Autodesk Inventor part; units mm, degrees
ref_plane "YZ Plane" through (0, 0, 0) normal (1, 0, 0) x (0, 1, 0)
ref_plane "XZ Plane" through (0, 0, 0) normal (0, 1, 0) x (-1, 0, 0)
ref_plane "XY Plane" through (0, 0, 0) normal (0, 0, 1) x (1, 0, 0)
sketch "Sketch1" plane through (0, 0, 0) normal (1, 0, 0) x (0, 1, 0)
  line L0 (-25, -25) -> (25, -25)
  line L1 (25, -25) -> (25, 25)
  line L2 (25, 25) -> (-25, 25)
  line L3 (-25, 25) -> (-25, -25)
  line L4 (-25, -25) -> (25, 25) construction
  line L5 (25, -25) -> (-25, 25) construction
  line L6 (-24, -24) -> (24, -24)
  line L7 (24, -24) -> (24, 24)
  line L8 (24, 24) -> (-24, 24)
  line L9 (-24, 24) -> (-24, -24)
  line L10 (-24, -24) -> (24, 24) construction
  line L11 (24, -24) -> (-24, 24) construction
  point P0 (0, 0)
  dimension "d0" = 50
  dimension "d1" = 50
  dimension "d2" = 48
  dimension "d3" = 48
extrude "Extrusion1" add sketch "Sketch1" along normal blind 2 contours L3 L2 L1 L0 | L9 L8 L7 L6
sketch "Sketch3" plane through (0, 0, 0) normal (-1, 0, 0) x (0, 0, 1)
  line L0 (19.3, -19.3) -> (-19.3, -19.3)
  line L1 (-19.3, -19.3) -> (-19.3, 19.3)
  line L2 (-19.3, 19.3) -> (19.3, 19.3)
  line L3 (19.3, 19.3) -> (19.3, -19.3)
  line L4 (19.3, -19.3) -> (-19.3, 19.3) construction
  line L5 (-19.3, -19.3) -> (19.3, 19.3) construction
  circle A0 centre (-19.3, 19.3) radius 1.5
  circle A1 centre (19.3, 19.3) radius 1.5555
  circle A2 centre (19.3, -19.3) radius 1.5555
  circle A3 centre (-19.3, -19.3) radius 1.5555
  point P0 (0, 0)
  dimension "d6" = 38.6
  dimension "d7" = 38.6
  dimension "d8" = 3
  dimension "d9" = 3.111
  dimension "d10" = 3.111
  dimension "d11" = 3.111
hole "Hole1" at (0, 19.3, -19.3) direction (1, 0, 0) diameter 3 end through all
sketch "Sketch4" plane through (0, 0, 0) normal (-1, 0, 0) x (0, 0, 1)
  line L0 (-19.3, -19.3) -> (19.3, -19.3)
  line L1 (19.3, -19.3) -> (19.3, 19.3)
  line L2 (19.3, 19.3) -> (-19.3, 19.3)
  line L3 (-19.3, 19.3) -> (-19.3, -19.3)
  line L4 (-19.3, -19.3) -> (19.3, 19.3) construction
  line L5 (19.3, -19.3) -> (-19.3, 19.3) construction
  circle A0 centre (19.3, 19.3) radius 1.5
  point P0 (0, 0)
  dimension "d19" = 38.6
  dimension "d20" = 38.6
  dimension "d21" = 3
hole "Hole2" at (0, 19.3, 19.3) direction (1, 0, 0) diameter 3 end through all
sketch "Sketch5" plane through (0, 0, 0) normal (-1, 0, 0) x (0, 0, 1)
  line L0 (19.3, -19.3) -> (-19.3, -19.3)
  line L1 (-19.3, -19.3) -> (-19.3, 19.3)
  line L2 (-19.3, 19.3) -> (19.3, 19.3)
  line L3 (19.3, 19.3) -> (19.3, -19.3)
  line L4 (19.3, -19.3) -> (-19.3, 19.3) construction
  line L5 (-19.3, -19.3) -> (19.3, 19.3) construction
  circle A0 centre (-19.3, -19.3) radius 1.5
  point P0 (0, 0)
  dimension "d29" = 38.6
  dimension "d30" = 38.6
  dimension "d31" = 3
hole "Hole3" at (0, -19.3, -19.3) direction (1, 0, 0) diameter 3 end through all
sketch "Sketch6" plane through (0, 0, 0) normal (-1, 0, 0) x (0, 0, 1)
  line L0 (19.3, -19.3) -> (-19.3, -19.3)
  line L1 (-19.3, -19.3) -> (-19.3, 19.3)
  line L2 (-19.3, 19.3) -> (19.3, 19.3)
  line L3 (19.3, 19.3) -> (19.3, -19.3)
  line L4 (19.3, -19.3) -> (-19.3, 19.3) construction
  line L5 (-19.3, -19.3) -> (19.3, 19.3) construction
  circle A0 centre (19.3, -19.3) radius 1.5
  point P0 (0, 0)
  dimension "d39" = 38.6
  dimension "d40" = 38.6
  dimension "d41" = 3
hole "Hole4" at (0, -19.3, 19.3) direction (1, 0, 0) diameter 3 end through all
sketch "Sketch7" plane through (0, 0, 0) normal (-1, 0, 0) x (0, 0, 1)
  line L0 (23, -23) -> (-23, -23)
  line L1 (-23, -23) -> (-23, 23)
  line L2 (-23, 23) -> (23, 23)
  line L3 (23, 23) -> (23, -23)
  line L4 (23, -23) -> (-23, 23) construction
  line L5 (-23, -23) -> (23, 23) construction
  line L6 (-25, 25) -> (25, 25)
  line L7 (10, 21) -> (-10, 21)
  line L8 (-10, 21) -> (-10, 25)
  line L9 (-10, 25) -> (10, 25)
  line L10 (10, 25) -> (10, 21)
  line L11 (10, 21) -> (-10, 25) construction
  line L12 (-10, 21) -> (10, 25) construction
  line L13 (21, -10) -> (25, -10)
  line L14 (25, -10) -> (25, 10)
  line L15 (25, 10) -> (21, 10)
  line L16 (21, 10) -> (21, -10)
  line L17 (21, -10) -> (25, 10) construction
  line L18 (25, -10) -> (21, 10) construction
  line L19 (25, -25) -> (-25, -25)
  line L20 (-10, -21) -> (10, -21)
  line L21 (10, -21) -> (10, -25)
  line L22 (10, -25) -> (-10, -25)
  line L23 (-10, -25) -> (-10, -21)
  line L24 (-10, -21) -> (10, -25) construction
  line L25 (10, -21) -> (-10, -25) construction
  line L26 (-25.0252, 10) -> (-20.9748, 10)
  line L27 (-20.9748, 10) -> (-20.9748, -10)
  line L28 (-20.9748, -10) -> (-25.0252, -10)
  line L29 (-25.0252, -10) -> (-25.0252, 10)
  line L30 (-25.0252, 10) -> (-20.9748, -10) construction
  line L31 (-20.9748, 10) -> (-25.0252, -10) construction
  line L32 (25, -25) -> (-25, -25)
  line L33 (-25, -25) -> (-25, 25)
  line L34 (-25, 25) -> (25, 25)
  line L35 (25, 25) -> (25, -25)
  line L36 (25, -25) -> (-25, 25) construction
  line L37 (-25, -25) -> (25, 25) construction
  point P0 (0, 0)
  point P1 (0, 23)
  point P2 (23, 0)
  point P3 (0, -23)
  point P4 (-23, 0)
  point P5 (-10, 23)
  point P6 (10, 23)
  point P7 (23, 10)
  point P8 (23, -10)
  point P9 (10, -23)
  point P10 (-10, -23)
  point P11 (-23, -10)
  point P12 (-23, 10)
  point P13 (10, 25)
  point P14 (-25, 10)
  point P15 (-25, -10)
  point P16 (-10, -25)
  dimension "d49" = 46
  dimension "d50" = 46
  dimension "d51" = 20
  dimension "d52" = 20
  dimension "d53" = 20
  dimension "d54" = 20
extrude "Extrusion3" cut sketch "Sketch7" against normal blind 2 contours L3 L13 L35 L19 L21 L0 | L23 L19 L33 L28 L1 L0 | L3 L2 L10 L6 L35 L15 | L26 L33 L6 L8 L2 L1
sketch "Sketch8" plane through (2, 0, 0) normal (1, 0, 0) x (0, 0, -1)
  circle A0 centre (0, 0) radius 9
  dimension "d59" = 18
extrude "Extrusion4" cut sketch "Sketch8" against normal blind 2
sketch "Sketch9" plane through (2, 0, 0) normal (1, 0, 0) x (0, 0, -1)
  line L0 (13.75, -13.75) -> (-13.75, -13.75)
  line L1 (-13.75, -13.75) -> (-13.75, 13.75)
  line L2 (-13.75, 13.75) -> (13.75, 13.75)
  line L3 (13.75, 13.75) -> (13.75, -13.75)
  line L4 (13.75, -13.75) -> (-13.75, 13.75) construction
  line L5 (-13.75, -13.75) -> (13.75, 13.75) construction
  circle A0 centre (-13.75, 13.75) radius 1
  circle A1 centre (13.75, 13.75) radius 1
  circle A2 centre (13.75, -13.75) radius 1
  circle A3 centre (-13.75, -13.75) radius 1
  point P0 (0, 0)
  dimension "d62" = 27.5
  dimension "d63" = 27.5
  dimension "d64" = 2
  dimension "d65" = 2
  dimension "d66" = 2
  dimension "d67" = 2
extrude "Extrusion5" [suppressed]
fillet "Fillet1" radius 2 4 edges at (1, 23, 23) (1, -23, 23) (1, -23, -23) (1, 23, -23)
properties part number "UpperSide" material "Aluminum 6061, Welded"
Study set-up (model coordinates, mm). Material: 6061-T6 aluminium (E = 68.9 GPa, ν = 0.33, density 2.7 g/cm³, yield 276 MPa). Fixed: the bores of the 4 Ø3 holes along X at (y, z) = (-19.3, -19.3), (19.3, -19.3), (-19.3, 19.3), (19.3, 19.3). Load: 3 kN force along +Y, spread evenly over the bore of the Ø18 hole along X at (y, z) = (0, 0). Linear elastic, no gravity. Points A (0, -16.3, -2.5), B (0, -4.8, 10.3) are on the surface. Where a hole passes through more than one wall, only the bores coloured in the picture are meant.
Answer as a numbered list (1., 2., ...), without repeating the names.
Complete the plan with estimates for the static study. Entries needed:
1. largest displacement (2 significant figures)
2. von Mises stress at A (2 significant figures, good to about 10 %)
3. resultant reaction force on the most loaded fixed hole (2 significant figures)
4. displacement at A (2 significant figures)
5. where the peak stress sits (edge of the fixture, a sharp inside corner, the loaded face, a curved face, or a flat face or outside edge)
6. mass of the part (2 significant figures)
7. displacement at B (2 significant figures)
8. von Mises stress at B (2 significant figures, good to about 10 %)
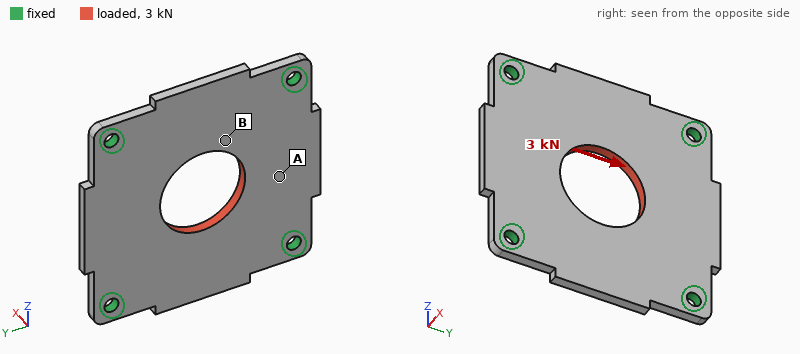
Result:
1. 15 µm
2. 14 MPa
3. 810 N
4. 13 µm
5. edge of the fixture
6. 11 g
7. 10.0 µm
8. 37 MPa
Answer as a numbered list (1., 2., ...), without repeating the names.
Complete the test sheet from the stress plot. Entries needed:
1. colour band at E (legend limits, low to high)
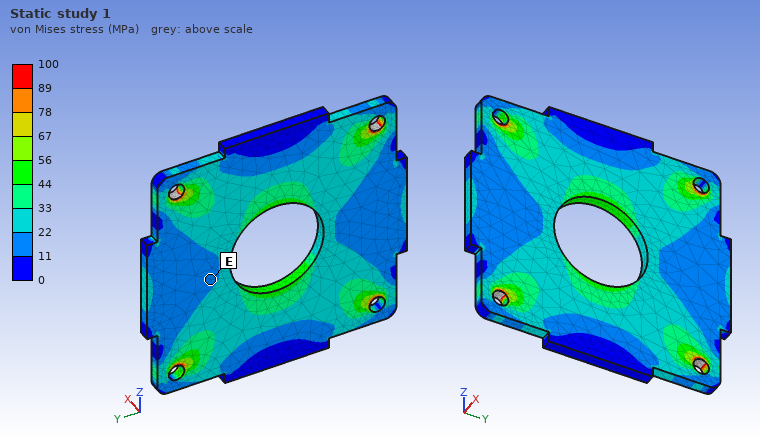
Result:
1. 11 to 22 MPa
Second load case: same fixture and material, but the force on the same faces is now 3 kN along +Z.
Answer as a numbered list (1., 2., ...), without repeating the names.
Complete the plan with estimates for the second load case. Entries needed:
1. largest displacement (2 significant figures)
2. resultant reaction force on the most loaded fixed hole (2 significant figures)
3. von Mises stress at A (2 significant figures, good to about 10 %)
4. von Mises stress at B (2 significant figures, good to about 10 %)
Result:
1. 15 µm
2. 810 N
3. 24 MPa
4. 24 MPa
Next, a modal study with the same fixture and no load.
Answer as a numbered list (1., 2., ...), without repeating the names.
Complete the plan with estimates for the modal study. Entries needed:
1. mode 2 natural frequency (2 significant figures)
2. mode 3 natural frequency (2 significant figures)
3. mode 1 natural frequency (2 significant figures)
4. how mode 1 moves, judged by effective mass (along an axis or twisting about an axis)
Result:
1. 7300 Hz
2. 7300 Hz
3. 5200 Hz
4. along X
